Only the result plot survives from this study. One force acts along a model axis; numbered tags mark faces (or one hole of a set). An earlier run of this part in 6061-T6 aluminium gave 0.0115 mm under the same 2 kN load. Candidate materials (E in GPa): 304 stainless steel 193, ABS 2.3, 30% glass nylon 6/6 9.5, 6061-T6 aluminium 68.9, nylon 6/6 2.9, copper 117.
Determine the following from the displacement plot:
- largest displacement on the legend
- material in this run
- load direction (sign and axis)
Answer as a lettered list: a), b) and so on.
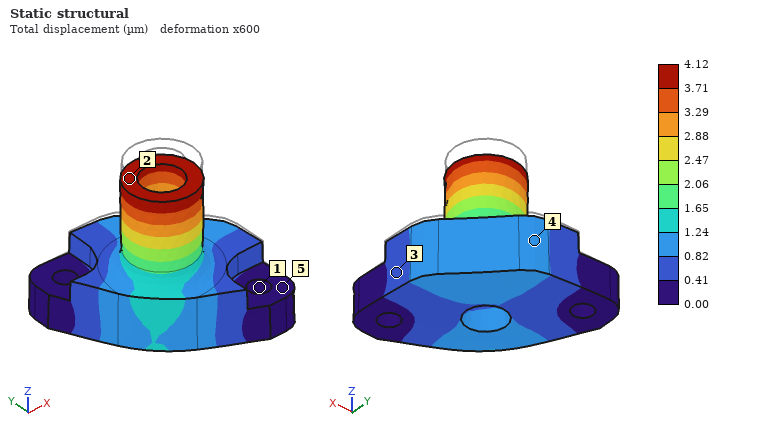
a) 4.12 µm
b) 304 stainless steel
c) -Z
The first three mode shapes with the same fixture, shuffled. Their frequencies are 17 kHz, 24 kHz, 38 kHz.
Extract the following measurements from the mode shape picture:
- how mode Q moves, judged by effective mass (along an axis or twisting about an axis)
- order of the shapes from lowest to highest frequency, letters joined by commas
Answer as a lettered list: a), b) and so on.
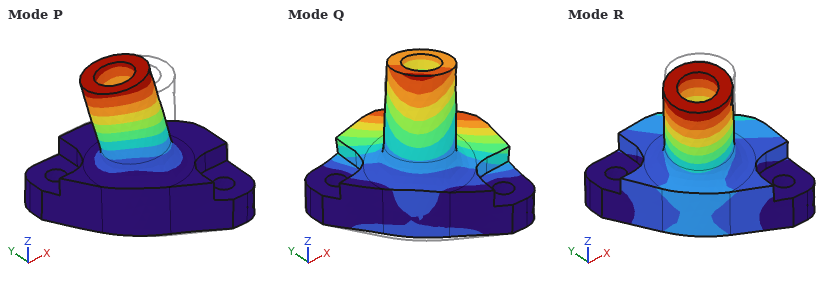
a) along Z
b) R, P, Q
